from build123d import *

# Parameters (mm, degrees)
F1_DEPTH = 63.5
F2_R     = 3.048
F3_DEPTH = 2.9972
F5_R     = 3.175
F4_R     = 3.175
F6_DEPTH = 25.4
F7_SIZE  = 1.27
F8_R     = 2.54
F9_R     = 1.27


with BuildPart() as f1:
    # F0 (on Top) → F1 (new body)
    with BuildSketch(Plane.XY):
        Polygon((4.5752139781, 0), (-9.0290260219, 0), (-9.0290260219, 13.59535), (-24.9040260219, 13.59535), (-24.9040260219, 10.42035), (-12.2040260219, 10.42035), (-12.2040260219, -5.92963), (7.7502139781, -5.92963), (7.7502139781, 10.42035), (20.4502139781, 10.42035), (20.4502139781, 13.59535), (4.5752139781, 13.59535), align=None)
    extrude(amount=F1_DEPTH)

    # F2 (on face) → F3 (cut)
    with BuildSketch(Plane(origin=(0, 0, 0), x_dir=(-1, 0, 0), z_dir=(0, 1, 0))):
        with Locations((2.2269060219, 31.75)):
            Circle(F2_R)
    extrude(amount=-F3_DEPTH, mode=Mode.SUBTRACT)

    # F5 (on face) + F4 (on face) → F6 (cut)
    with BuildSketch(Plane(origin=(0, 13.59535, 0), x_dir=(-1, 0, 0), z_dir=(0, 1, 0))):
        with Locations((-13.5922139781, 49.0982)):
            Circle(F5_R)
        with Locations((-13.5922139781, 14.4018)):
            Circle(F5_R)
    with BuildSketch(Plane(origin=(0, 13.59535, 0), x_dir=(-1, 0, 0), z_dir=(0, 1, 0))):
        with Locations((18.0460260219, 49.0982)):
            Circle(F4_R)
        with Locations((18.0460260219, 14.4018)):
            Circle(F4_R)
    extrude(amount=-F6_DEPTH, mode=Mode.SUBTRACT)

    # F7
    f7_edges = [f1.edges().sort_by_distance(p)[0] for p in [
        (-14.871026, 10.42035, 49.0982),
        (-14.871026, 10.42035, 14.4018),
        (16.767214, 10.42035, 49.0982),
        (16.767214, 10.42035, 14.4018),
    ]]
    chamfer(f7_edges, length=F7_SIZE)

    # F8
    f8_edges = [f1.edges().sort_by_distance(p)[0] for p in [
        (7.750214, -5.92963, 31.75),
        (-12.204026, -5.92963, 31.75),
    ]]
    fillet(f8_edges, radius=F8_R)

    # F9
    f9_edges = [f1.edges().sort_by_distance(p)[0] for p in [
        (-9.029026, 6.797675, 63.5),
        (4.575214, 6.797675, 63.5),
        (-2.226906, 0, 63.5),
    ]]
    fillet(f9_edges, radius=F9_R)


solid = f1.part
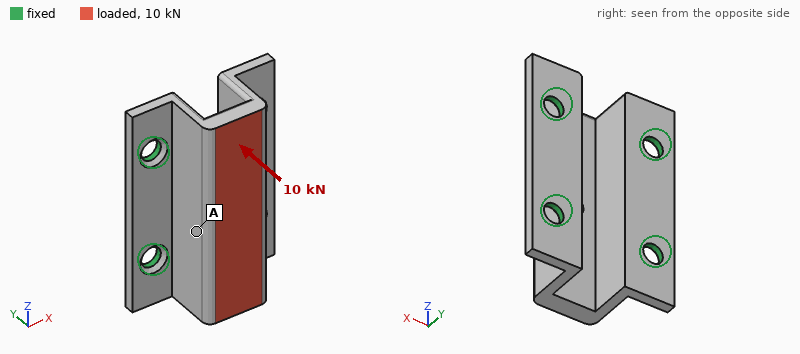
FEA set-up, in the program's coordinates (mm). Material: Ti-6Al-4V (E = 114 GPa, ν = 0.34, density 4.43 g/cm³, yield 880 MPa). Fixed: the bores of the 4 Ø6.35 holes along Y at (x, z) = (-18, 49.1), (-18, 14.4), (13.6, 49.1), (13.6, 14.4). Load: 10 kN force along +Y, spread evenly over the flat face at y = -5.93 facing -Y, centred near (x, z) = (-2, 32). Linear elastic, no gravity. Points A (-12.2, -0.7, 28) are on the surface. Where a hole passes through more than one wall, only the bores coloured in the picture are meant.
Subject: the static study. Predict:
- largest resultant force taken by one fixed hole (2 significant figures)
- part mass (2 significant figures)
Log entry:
2.7 kN
77 g
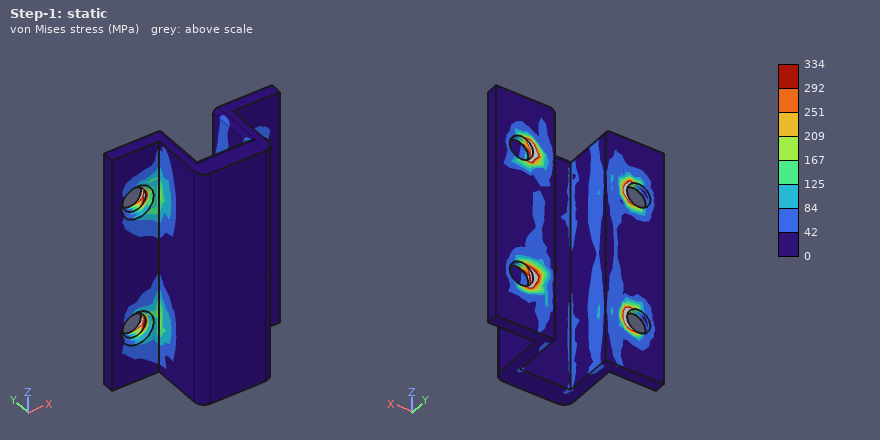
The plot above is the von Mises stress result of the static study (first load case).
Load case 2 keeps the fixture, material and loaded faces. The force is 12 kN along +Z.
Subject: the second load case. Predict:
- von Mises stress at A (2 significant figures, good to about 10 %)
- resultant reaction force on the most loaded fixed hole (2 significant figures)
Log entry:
62 MPa
4.6 kN
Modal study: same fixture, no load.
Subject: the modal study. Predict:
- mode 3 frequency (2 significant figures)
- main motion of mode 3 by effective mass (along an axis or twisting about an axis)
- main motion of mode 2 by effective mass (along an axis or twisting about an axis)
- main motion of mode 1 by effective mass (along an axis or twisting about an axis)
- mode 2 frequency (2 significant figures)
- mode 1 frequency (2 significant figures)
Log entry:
11 kHz
twisting about Y
along Z
along X
9900 Hz
8800 Hz
